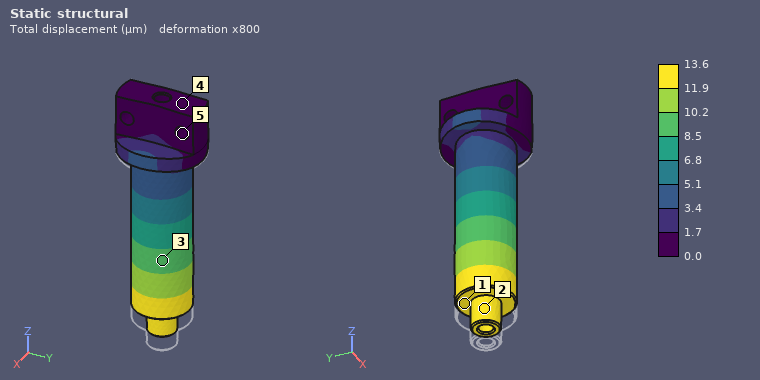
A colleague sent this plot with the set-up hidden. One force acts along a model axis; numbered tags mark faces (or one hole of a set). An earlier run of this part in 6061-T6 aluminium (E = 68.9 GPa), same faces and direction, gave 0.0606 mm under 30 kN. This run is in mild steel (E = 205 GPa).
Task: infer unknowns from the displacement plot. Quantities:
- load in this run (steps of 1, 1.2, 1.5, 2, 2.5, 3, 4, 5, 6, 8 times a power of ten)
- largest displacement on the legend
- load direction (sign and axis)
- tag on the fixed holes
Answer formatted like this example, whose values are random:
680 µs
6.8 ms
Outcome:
20 kN
13.6 µm
+Z
5
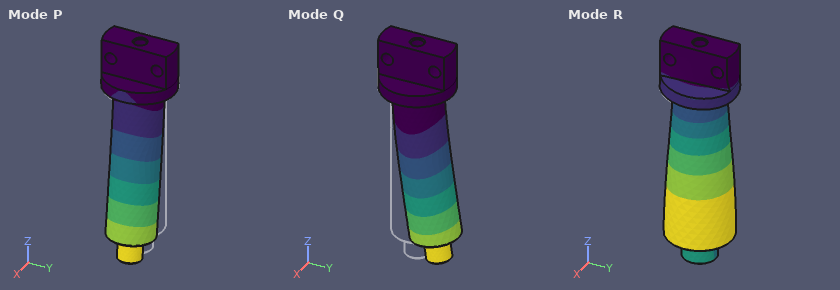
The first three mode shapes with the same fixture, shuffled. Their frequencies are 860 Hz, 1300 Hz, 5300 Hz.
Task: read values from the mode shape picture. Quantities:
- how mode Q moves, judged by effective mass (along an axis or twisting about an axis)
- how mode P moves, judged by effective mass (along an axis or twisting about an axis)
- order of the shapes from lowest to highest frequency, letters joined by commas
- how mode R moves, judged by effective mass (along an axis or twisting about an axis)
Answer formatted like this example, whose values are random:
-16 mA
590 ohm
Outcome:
along Y
along X
P, Q, R
twisting about Z
